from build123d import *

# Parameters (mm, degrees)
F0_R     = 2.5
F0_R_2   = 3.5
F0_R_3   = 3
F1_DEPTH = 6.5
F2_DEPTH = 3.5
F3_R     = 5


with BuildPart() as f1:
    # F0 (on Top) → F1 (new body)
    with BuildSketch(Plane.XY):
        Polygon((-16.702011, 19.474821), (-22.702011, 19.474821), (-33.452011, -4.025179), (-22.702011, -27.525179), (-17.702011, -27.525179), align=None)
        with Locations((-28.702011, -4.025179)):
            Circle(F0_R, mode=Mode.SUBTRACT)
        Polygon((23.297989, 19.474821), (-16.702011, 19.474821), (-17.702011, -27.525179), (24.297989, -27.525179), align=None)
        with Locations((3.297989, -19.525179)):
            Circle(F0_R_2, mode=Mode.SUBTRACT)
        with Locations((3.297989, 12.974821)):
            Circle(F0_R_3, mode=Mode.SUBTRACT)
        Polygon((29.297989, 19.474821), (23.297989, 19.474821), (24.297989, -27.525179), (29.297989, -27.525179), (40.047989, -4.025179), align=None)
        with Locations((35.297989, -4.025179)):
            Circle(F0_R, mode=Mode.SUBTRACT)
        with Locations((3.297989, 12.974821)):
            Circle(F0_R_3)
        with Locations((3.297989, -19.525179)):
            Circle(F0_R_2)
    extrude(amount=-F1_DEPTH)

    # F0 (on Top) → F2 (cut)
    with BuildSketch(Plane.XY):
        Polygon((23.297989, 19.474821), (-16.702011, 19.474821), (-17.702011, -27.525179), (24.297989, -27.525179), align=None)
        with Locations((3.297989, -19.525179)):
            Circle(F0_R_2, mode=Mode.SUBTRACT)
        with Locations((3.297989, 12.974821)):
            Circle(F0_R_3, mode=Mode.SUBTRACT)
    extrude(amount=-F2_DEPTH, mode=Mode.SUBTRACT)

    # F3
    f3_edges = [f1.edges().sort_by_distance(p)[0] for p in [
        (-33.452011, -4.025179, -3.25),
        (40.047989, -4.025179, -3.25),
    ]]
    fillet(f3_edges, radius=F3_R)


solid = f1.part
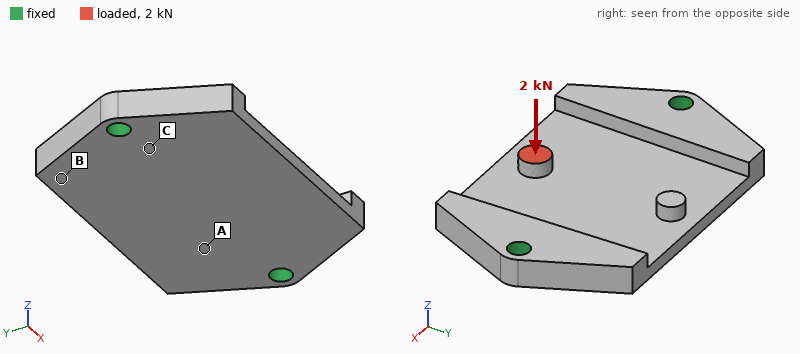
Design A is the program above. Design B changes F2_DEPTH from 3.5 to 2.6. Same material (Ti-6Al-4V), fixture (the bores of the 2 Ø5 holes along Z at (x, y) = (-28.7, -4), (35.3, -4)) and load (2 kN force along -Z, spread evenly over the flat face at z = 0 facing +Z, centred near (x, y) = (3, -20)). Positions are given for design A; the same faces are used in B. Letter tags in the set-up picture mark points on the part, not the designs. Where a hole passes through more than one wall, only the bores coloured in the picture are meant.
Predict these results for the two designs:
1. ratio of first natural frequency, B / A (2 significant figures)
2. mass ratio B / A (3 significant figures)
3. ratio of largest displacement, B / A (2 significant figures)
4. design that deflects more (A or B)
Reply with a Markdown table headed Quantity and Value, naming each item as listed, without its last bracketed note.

| Quantity | Value |
|---|---|
| ratio of first natural frequency, B / A | 1.00 |
| mass ratio B / A | 1.14 |
| ratio of largest displacement, B / A | 0.69 |
| design that deflects more | A |
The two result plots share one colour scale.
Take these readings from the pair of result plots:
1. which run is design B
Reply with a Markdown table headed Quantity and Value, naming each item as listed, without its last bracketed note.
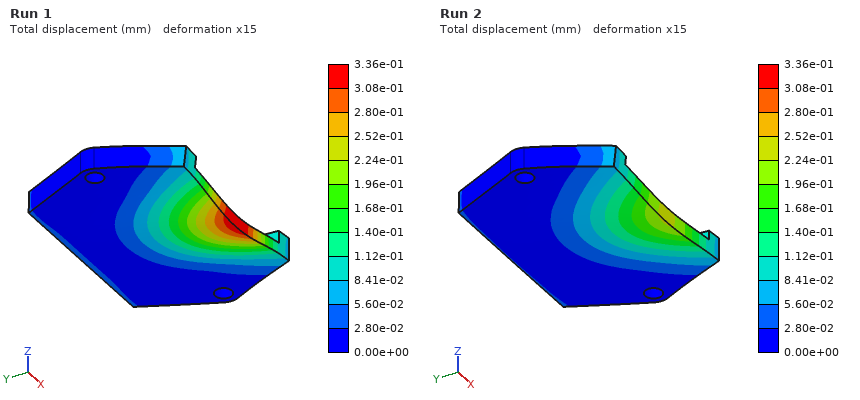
| Quantity | Value |
|---|---|
| which run is design B | Run 2 |
